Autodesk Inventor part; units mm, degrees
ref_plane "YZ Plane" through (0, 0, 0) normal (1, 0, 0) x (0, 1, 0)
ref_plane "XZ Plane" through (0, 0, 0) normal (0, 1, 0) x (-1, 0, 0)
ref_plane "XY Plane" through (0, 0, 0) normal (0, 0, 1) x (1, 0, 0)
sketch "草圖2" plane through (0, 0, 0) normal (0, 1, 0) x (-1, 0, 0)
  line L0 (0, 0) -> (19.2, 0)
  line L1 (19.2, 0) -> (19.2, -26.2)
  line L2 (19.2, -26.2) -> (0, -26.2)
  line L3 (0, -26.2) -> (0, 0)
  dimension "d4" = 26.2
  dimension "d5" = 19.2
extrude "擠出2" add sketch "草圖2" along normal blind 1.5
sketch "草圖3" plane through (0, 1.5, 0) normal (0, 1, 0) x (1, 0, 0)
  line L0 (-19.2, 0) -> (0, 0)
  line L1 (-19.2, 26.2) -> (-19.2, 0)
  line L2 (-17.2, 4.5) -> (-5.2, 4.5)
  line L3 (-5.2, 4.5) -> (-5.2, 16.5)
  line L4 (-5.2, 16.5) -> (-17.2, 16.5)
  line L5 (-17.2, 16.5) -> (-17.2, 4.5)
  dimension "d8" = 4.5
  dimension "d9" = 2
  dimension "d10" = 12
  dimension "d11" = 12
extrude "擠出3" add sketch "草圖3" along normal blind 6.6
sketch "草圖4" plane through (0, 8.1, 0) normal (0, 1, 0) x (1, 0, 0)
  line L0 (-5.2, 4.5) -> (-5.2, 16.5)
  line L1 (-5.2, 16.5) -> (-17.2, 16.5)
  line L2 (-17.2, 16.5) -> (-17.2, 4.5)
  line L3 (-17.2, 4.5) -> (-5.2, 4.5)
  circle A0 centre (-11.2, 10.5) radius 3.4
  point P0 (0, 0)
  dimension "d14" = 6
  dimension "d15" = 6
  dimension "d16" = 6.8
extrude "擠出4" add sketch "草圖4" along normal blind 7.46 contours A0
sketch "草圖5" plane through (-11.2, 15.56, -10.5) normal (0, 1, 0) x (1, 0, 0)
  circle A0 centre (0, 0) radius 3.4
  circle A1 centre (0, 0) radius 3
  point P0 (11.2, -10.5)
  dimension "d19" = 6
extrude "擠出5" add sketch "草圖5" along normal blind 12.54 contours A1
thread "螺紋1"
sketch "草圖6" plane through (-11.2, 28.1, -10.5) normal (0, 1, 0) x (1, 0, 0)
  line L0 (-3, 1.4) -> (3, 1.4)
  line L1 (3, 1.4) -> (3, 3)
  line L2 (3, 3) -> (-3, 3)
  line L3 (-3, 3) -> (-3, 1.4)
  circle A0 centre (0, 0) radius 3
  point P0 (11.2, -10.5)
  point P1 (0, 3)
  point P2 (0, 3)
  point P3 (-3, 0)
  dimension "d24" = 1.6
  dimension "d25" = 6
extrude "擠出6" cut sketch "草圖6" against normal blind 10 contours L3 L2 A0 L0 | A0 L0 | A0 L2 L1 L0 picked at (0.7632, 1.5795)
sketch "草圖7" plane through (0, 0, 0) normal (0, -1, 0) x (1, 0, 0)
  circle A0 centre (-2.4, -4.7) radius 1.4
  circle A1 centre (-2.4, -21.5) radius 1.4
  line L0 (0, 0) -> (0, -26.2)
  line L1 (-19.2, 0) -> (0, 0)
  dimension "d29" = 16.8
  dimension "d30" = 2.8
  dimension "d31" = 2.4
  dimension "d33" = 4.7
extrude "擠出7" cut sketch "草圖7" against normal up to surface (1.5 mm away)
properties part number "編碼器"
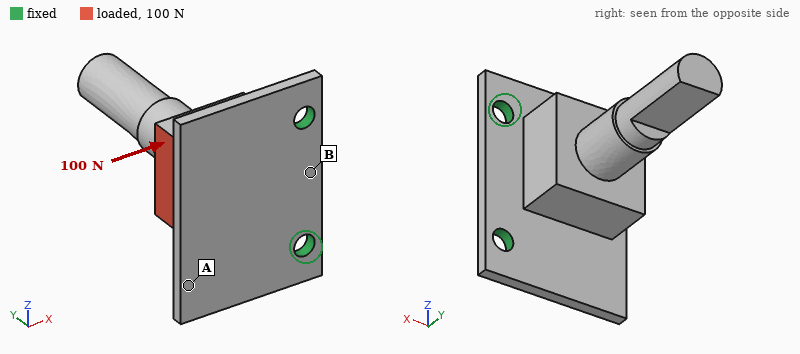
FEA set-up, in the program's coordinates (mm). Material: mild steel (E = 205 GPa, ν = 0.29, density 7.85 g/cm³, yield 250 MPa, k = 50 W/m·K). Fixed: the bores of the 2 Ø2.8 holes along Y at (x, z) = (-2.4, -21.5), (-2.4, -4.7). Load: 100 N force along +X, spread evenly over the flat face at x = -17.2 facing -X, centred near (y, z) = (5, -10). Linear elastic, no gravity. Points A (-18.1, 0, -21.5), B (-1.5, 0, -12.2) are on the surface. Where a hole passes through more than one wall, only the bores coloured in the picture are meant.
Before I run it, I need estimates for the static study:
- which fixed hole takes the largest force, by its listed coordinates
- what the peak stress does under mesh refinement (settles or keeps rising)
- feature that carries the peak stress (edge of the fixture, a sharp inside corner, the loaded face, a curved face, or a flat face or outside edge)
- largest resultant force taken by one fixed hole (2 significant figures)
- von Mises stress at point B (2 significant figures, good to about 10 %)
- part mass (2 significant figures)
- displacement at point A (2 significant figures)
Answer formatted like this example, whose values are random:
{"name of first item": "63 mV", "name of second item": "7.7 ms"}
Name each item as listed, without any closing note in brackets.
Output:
{"which fixed hole takes the largest force, by its listed coordinates": "(-2.4, -4.7)", "what the peak stress does under mesh refinement": "keeps rising", "feature that carries the peak stress": "edge of the fixture", "largest resultant force taken by one fixed hole": "68 N", "von Mises stress at point B": "15 MPa", "part mass": "18 g", "displacement at point A": "14 µm"}
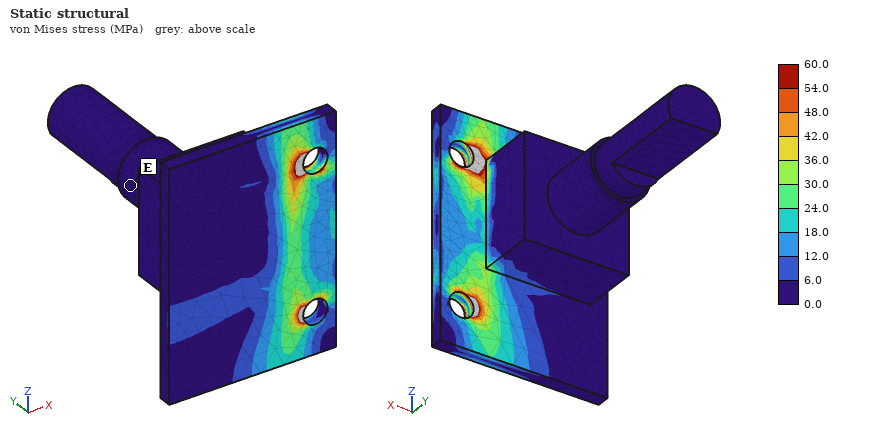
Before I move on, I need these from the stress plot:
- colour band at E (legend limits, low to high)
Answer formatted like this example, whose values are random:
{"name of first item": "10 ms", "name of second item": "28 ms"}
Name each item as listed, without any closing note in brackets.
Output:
{"colour band at E": "0.0 to 6.0 MPa"}
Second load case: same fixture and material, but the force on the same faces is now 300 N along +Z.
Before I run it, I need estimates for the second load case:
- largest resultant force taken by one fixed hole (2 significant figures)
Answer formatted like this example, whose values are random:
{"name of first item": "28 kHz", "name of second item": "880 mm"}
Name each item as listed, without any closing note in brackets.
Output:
{"largest resultant force taken by one fixed hole": "300 N"}
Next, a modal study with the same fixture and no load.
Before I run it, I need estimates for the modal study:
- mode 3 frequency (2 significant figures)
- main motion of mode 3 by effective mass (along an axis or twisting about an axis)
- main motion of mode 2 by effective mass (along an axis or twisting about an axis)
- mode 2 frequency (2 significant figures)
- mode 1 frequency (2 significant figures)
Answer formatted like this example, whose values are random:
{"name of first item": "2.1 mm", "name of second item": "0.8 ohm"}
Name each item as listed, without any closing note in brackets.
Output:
{"mode 3 frequency": "12 kHz", "main motion of mode 3 by effective mass": "along Y", "main motion of mode 2 by effective mass": "along Z", "mode 2 frequency": "5700 Hz", "mode 1 frequency": "1900 Hz"}
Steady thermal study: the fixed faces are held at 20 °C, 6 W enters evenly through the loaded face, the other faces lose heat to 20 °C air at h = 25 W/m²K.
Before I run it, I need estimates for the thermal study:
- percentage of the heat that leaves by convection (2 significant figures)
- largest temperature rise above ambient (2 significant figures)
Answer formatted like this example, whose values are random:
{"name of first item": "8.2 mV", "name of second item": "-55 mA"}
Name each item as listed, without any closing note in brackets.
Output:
{"percentage of the heat that leaves by convection": "14 %", "largest temperature rise above ambient": "31 K"}
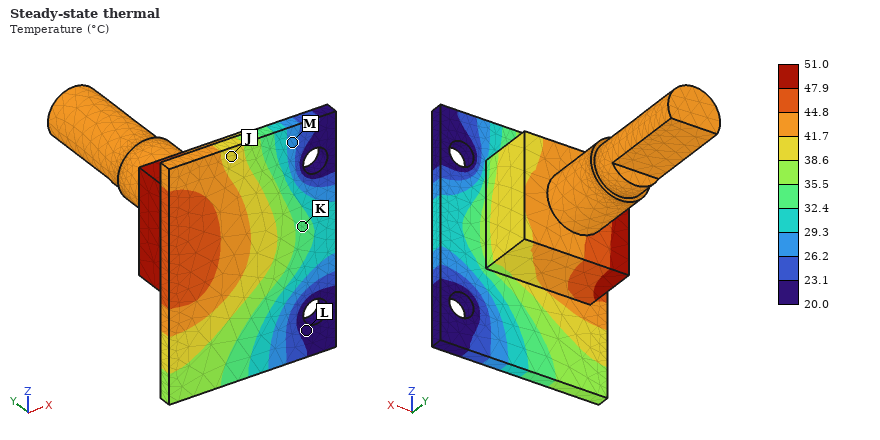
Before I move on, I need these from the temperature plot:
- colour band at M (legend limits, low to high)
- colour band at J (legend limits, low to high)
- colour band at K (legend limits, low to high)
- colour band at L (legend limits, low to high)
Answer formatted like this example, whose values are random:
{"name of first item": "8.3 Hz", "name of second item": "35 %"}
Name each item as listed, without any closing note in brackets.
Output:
{"colour band at M": "26.2 to 29.3 °C", "colour band at J": "38.6 to 41.7 °C", "colour band at K": "32.4 to 35.5 °C", "colour band at L": "20.0 to 23.1 °C"}
